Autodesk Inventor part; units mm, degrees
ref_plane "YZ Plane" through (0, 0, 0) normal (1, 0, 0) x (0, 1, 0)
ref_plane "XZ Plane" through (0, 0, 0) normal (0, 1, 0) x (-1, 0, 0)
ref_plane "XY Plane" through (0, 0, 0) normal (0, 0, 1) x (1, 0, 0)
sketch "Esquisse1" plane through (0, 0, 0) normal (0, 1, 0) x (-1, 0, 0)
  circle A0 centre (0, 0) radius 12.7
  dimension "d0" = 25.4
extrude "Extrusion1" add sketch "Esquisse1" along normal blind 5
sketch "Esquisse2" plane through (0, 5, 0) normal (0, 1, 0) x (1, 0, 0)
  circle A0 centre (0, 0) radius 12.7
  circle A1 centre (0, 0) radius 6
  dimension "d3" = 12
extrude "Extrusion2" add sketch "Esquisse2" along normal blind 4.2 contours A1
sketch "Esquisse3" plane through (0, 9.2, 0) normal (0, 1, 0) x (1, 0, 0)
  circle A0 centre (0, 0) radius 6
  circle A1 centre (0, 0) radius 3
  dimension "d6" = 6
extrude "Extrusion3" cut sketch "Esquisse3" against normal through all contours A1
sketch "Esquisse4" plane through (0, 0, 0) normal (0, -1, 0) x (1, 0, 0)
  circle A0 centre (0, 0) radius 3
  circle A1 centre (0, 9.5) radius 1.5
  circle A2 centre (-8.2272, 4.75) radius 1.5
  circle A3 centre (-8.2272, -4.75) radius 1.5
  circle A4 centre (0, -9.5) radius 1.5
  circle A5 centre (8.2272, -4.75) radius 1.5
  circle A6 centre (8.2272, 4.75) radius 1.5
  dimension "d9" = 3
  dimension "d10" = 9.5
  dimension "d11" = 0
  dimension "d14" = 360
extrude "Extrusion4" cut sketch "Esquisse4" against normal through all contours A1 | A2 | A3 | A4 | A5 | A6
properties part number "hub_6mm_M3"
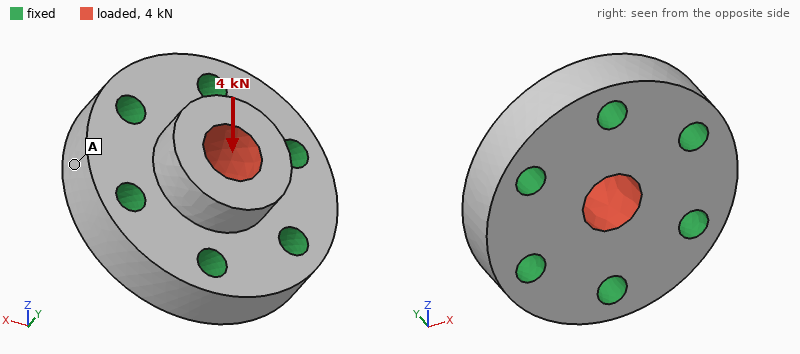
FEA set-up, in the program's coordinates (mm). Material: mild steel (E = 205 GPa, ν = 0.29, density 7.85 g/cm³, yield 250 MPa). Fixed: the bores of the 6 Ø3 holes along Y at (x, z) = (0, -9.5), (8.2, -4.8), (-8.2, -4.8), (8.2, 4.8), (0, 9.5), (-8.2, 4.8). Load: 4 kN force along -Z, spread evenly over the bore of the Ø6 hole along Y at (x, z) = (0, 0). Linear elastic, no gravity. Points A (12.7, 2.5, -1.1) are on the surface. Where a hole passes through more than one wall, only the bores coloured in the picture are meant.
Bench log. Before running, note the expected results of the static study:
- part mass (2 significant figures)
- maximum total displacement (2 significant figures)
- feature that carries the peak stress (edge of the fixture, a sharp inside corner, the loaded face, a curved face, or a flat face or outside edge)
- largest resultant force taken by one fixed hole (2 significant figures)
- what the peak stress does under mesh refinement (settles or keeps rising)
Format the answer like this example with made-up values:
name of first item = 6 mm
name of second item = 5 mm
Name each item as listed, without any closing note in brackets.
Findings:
part mass = 20 g
maximum total displacement = 2.8 µm
feature that carries the peak stress = a sharp inside corner
largest resultant force taken by one fixed hole = 1.1 kN
what the peak stress does under mesh refinement = keeps rising
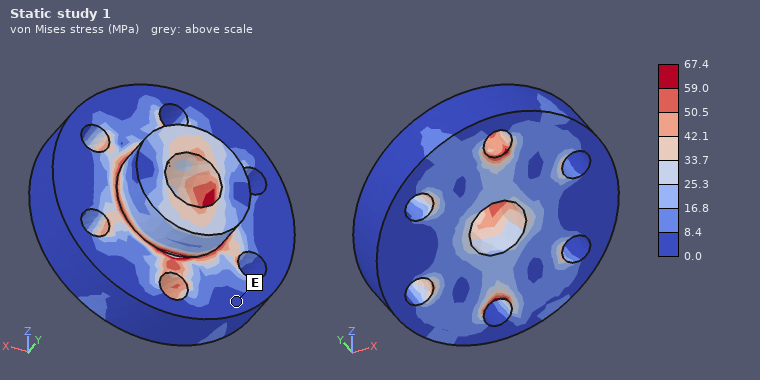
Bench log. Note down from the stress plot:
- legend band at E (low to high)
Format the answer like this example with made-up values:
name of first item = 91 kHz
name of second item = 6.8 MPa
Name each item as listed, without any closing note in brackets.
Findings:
legend band at E = 0.0 to 8.4 MPa
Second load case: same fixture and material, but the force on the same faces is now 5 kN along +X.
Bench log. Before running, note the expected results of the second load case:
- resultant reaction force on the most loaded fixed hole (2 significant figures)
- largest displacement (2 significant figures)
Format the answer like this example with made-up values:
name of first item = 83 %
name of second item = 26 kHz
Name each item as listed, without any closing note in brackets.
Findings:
resultant reaction force on the most loaded fixed hole = 1.2 kN
largest displacement = 3.5 µm
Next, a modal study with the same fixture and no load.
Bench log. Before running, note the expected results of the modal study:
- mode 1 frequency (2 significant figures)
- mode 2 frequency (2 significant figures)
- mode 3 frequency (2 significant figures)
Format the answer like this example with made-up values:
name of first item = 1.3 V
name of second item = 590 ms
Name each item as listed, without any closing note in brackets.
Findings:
mode 1 frequency = 93 kHz
mode 2 frequency = 96 kHz
mode 3 frequency = 96 kHz
